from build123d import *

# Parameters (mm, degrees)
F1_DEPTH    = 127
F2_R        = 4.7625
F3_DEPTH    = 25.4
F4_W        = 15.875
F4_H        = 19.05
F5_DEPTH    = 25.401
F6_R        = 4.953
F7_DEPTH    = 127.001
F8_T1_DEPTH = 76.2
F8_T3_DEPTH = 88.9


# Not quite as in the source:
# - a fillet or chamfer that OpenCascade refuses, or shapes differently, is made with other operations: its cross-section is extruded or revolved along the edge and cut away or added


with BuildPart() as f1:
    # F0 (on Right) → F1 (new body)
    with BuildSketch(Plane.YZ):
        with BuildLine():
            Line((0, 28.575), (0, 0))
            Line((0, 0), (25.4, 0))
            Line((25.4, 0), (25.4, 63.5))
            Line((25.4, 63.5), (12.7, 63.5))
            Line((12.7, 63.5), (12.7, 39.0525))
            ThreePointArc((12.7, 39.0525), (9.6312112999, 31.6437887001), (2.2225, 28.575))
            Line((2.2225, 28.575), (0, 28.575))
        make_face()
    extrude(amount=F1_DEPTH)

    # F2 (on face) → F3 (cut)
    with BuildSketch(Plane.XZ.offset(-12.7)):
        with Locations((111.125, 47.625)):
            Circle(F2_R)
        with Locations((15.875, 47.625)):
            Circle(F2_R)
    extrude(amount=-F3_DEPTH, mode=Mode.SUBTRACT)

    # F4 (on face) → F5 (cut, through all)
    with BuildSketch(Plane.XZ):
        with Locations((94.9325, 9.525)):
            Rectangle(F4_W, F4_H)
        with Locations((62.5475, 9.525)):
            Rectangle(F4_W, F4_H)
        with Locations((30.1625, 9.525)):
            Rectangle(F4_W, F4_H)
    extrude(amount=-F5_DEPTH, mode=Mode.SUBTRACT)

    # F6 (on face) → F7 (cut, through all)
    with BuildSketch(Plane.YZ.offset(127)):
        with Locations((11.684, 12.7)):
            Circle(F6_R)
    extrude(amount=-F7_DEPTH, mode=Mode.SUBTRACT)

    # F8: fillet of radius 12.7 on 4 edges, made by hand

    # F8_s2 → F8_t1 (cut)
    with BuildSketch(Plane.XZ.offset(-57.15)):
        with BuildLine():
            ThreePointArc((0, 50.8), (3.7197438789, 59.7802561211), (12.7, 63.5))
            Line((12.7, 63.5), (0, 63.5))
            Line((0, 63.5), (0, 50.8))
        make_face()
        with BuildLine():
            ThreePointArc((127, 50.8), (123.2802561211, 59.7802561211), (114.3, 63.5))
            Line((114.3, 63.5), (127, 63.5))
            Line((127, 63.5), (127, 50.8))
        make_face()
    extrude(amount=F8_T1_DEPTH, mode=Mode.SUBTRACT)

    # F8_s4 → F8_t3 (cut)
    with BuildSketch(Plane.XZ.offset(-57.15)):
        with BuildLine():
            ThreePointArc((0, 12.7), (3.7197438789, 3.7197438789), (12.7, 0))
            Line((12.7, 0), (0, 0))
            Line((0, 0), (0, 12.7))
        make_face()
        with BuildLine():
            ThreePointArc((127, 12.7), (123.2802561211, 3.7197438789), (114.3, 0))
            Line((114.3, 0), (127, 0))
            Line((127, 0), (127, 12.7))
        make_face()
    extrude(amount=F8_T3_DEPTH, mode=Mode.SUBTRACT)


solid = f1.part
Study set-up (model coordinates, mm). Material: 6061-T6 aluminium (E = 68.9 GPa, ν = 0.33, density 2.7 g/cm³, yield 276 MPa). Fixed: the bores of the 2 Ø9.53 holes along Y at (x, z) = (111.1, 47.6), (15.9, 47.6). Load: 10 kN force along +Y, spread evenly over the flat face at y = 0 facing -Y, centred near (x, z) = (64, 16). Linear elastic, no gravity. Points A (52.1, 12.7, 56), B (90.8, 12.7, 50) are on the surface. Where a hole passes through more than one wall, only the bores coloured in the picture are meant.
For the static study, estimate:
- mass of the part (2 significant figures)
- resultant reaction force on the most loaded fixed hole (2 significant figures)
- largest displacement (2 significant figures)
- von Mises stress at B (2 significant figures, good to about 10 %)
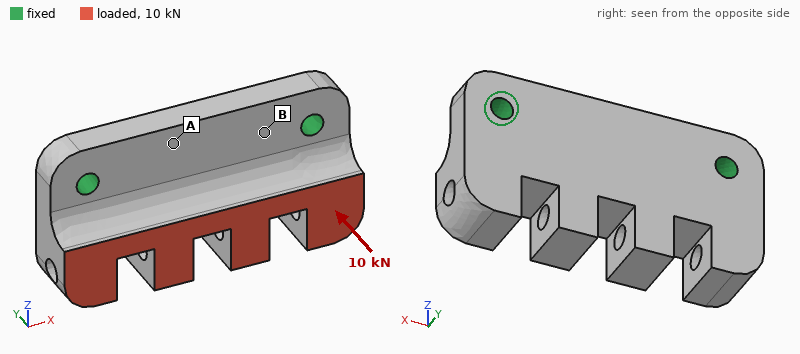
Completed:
320 g
5.1 kN
0.23 mm
41 MPa
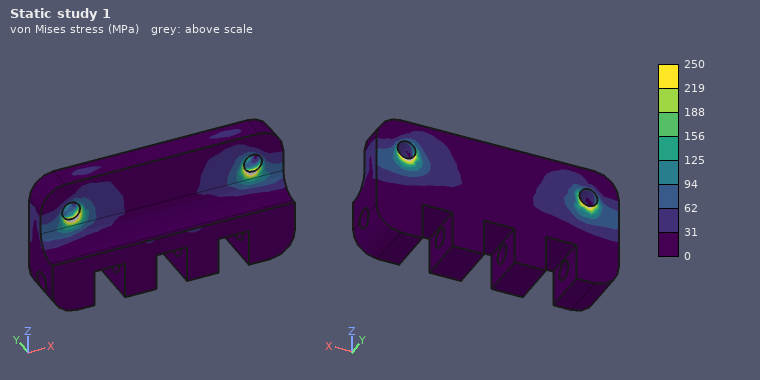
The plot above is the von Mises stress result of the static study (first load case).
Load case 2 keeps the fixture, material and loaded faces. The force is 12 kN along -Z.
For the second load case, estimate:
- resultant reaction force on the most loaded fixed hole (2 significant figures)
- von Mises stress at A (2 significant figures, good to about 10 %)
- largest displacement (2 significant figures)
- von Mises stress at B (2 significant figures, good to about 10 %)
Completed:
6.2 kN
17 MPa
0.21 mm
44 MPa
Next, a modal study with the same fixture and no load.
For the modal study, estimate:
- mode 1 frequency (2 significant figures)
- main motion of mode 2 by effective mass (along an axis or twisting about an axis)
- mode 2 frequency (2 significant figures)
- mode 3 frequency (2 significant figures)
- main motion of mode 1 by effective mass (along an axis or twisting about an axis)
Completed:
3100 Hz
twisting about Z
4800 Hz
6300 Hz
along Y
